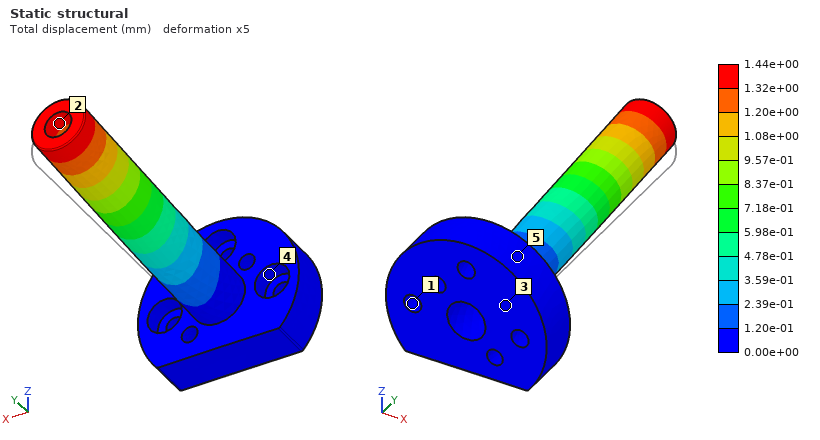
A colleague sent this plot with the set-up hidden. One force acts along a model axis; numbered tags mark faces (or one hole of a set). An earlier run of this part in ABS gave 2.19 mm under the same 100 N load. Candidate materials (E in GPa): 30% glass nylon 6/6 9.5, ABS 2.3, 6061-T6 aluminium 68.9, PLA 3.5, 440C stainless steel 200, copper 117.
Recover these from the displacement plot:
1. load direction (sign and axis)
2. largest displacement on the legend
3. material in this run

+Z
1.44e+00 mm
PLA
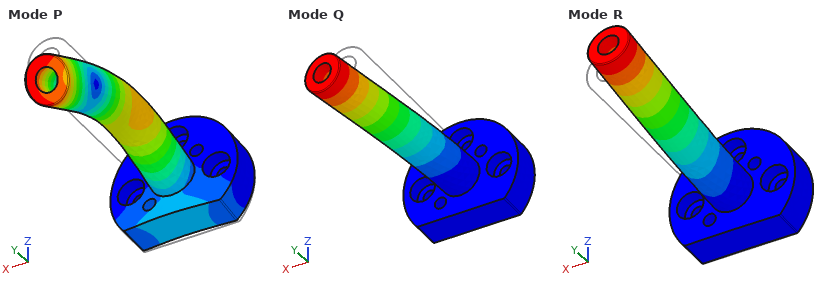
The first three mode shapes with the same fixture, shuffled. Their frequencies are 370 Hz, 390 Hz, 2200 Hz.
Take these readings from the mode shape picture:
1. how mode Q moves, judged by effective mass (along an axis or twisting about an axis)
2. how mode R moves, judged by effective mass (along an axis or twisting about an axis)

along X
along Z
